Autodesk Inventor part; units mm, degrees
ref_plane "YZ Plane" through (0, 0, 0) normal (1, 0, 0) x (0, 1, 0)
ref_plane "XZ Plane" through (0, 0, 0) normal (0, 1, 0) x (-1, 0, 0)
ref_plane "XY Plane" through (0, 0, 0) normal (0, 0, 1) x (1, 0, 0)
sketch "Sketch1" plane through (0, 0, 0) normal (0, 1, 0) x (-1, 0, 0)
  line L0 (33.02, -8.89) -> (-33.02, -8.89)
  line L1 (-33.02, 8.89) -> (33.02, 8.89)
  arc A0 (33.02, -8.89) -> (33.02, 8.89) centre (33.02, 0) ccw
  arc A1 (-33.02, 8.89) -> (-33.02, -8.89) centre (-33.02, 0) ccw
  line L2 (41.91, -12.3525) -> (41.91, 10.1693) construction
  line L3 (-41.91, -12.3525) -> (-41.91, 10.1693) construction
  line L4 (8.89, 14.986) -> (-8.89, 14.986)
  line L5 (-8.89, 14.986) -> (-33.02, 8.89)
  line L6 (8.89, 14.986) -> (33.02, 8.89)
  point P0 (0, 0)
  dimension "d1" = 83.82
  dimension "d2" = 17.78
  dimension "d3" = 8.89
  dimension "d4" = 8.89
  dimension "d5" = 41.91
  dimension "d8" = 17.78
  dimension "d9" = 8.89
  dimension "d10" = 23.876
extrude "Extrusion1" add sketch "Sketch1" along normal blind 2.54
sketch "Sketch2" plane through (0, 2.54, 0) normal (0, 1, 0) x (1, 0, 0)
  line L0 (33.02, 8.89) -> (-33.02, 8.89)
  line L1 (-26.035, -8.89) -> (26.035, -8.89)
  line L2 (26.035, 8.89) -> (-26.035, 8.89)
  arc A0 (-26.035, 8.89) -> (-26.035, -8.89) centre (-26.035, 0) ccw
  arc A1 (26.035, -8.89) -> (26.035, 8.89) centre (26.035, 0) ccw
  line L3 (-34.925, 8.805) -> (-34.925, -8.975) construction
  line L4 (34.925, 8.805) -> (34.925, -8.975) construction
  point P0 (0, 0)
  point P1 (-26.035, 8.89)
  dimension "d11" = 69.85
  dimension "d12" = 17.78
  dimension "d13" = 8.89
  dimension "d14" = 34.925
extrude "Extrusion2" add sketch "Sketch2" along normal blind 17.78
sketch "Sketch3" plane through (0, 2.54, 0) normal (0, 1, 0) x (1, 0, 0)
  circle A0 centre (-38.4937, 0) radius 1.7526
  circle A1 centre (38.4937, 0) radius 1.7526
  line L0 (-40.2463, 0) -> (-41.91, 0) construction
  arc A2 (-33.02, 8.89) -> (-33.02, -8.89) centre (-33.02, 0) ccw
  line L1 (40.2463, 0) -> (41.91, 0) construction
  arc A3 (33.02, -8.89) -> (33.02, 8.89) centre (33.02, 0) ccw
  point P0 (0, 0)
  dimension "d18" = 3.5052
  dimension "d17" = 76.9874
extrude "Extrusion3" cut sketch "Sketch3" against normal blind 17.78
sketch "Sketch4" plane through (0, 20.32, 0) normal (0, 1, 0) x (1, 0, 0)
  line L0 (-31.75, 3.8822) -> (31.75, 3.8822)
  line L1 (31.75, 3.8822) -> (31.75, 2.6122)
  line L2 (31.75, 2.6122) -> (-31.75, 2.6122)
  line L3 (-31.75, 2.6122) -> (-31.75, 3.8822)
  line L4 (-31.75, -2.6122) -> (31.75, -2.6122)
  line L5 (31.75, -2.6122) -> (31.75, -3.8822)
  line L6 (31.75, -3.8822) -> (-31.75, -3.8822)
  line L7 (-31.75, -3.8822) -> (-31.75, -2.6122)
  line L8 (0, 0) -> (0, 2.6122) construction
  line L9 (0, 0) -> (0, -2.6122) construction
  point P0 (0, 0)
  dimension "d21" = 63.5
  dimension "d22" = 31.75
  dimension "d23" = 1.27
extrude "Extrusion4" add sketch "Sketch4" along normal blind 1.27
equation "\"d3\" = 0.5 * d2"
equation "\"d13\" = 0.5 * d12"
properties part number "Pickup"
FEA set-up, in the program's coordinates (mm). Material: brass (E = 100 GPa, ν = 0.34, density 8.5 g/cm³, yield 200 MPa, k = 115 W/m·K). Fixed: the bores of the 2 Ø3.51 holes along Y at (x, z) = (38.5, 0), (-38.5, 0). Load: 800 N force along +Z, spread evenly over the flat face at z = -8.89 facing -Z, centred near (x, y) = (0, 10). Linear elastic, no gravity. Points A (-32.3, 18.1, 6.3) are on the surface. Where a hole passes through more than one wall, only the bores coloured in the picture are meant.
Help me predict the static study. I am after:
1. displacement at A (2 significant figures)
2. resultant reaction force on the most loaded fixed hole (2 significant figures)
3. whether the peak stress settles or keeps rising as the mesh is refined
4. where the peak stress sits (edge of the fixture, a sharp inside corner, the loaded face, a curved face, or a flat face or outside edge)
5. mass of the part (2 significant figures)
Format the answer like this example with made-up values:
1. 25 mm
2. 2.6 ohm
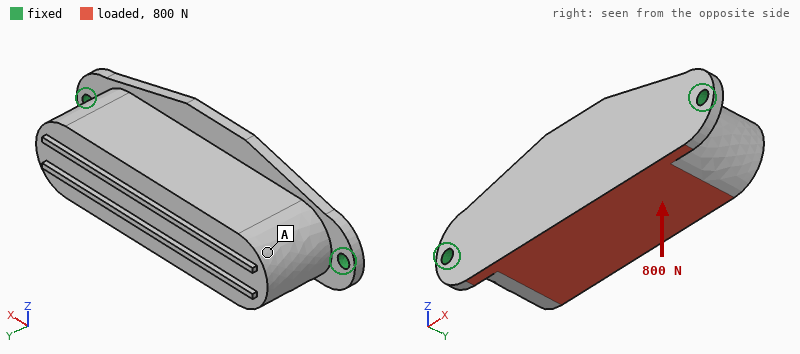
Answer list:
1. 78 µm
2. 400 N
3. keeps rising
4. edge of the fixture
5. 210 g
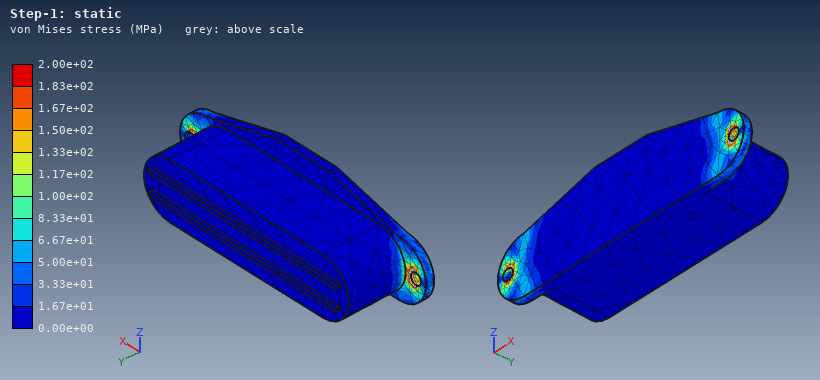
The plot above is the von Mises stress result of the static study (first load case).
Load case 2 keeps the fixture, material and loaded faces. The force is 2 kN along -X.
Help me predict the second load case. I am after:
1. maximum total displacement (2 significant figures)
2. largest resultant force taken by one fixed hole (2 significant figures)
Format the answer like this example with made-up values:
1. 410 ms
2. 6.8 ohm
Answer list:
1. 5.9 µm
2. 1.1 kN
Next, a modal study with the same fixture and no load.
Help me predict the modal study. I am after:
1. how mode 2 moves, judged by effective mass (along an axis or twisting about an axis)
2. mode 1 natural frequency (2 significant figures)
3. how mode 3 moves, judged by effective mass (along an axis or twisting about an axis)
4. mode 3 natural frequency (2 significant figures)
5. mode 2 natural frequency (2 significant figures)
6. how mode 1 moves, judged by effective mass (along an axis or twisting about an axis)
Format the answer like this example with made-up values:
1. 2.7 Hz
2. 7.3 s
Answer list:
1. along Y
2. 1200 Hz
3. along Z
4. 5700 Hz
5. 4100 Hz
6. along Z
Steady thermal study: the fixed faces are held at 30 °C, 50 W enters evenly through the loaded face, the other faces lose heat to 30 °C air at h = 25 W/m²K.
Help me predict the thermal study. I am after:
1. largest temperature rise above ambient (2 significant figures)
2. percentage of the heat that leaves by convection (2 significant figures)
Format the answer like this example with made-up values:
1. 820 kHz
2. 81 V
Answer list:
1. 50 K
2. 12 %
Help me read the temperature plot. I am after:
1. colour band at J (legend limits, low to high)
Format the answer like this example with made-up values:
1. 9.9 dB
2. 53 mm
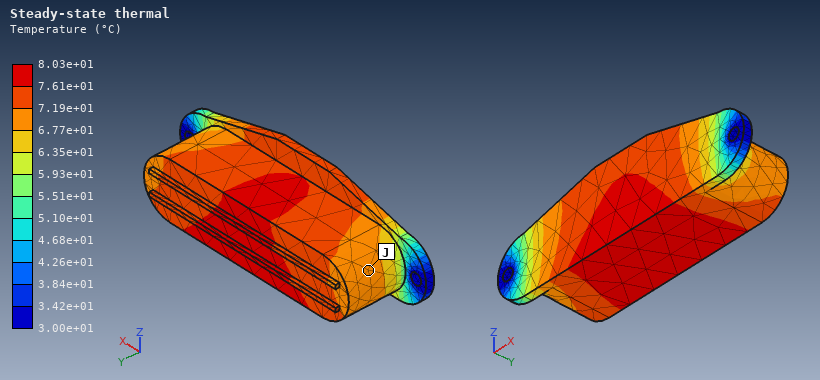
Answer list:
1. 6.77e+01 to 7.19e+01 °C
